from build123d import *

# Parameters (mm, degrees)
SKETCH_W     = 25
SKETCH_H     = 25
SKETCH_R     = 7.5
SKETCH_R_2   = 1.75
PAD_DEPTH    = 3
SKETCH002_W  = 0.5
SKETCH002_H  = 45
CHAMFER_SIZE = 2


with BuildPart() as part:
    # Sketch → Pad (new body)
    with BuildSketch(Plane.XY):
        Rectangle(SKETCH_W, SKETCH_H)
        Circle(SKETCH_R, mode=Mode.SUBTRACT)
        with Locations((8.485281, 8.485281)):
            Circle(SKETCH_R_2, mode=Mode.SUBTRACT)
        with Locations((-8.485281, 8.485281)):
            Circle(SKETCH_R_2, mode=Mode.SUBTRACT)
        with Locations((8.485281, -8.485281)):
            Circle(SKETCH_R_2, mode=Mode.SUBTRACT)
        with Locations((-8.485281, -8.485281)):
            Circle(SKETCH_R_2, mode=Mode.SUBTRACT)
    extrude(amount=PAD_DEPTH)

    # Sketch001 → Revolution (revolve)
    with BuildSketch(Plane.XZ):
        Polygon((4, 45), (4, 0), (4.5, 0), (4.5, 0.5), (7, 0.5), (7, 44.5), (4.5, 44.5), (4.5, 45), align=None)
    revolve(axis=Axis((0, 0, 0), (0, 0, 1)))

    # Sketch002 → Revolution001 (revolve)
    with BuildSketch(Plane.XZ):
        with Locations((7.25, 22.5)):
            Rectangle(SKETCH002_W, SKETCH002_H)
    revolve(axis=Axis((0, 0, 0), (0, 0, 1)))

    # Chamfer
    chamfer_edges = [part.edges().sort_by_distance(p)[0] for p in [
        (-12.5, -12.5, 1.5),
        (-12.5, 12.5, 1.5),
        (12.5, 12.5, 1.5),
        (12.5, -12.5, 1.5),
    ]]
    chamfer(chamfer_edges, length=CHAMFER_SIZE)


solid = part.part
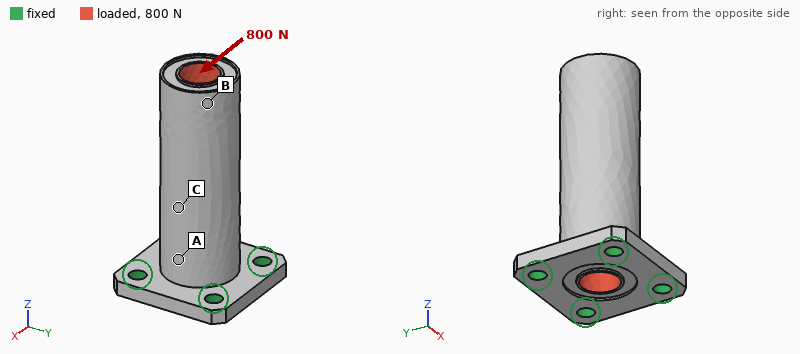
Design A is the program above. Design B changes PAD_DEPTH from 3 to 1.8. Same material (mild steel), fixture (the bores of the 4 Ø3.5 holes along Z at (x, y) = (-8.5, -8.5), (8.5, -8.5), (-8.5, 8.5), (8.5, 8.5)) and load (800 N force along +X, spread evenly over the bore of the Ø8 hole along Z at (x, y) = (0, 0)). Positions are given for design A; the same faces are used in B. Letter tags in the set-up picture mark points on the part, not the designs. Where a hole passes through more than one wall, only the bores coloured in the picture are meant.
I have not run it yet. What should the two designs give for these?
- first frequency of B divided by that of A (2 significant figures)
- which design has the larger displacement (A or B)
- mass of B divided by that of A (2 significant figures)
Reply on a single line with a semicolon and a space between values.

0.71; B; 0.93
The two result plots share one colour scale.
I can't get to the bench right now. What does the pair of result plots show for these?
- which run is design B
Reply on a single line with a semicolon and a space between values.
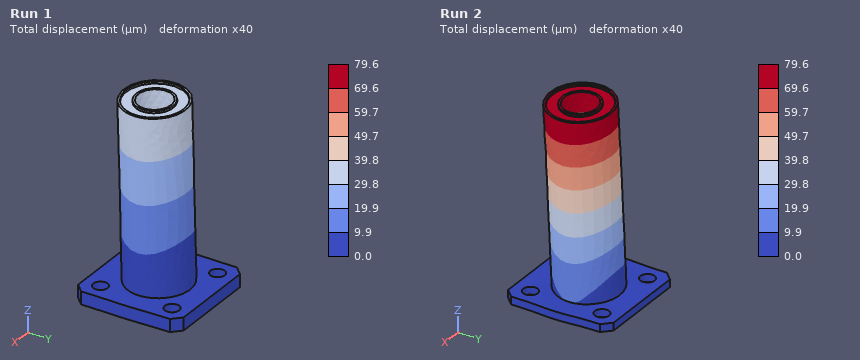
Run 2
